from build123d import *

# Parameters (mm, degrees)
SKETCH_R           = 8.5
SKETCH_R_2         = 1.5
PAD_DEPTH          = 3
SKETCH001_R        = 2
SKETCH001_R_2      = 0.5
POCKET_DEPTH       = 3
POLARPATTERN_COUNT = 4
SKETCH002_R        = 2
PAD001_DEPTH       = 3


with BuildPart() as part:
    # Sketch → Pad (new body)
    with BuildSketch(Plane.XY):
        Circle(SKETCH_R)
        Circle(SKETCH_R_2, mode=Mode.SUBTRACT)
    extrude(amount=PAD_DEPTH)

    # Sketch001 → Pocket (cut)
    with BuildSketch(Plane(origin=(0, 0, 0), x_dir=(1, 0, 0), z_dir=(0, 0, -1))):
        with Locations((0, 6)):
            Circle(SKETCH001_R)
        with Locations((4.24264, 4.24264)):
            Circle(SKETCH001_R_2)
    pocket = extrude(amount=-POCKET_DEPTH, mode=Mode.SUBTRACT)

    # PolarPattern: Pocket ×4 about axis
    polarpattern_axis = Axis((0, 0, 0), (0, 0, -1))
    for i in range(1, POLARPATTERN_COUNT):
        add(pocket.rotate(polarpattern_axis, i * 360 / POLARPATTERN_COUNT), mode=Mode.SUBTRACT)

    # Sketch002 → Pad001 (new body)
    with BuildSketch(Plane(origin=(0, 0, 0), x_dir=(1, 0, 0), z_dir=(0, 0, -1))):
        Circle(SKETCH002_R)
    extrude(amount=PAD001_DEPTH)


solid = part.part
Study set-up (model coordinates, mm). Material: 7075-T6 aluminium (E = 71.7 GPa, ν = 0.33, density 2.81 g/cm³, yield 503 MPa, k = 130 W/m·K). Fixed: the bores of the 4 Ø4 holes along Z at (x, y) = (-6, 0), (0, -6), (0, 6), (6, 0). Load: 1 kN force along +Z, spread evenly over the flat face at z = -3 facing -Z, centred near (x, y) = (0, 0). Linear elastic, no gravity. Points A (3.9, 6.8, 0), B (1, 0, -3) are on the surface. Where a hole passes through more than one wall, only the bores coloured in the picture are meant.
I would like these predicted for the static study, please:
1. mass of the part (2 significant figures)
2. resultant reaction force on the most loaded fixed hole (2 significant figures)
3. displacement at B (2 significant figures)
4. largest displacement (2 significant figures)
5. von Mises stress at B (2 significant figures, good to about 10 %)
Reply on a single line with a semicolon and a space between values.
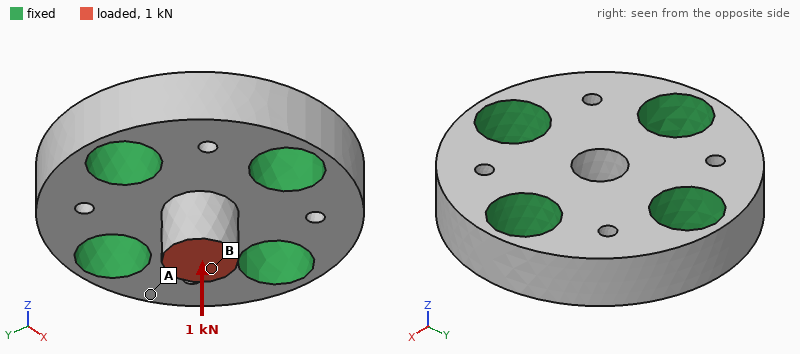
1.5 g; 280 N; 7.8 µm; 7.8 µm; 81 MPa
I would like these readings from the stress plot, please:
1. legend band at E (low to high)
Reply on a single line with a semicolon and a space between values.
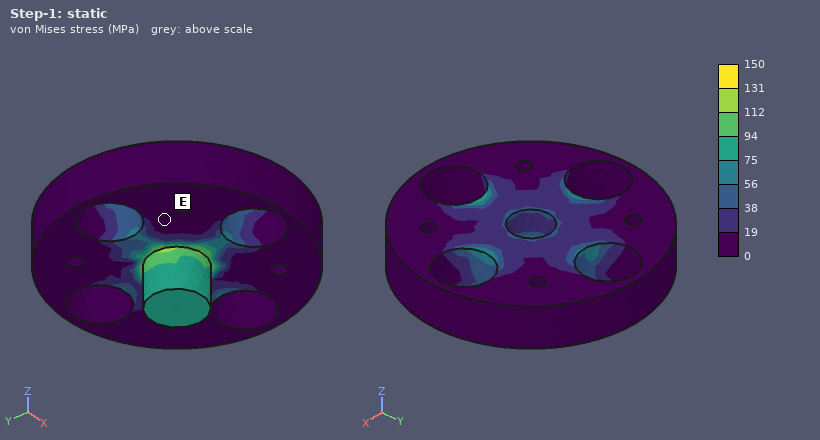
0 to 19 MPa
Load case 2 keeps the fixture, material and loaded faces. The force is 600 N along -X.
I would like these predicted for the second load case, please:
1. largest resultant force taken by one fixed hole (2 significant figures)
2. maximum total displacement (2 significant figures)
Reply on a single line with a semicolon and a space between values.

410 N; 26 µm
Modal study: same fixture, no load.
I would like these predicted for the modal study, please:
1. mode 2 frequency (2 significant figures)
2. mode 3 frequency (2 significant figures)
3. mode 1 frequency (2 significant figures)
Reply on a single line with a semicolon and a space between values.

120 kHz; 160 kHz; 120 kHz
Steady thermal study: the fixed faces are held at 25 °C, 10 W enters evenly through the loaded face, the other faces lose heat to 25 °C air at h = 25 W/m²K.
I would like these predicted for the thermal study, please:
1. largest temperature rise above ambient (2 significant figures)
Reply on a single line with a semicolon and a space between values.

31 K
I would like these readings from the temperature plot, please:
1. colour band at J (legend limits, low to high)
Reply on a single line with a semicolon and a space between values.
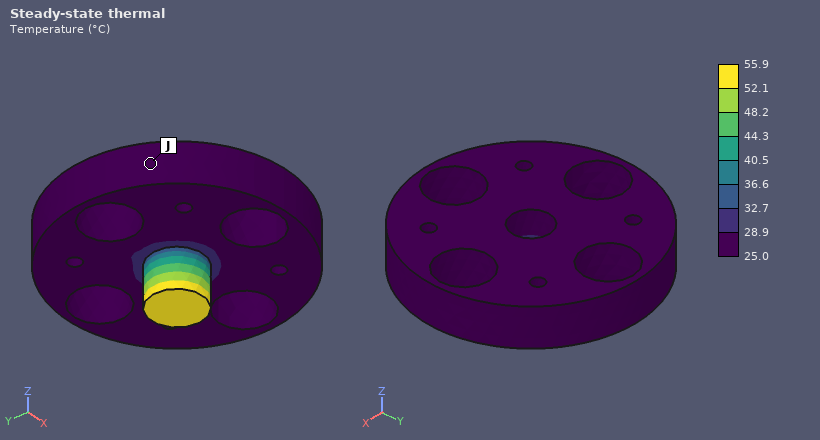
25.0 to 28.9 °C
